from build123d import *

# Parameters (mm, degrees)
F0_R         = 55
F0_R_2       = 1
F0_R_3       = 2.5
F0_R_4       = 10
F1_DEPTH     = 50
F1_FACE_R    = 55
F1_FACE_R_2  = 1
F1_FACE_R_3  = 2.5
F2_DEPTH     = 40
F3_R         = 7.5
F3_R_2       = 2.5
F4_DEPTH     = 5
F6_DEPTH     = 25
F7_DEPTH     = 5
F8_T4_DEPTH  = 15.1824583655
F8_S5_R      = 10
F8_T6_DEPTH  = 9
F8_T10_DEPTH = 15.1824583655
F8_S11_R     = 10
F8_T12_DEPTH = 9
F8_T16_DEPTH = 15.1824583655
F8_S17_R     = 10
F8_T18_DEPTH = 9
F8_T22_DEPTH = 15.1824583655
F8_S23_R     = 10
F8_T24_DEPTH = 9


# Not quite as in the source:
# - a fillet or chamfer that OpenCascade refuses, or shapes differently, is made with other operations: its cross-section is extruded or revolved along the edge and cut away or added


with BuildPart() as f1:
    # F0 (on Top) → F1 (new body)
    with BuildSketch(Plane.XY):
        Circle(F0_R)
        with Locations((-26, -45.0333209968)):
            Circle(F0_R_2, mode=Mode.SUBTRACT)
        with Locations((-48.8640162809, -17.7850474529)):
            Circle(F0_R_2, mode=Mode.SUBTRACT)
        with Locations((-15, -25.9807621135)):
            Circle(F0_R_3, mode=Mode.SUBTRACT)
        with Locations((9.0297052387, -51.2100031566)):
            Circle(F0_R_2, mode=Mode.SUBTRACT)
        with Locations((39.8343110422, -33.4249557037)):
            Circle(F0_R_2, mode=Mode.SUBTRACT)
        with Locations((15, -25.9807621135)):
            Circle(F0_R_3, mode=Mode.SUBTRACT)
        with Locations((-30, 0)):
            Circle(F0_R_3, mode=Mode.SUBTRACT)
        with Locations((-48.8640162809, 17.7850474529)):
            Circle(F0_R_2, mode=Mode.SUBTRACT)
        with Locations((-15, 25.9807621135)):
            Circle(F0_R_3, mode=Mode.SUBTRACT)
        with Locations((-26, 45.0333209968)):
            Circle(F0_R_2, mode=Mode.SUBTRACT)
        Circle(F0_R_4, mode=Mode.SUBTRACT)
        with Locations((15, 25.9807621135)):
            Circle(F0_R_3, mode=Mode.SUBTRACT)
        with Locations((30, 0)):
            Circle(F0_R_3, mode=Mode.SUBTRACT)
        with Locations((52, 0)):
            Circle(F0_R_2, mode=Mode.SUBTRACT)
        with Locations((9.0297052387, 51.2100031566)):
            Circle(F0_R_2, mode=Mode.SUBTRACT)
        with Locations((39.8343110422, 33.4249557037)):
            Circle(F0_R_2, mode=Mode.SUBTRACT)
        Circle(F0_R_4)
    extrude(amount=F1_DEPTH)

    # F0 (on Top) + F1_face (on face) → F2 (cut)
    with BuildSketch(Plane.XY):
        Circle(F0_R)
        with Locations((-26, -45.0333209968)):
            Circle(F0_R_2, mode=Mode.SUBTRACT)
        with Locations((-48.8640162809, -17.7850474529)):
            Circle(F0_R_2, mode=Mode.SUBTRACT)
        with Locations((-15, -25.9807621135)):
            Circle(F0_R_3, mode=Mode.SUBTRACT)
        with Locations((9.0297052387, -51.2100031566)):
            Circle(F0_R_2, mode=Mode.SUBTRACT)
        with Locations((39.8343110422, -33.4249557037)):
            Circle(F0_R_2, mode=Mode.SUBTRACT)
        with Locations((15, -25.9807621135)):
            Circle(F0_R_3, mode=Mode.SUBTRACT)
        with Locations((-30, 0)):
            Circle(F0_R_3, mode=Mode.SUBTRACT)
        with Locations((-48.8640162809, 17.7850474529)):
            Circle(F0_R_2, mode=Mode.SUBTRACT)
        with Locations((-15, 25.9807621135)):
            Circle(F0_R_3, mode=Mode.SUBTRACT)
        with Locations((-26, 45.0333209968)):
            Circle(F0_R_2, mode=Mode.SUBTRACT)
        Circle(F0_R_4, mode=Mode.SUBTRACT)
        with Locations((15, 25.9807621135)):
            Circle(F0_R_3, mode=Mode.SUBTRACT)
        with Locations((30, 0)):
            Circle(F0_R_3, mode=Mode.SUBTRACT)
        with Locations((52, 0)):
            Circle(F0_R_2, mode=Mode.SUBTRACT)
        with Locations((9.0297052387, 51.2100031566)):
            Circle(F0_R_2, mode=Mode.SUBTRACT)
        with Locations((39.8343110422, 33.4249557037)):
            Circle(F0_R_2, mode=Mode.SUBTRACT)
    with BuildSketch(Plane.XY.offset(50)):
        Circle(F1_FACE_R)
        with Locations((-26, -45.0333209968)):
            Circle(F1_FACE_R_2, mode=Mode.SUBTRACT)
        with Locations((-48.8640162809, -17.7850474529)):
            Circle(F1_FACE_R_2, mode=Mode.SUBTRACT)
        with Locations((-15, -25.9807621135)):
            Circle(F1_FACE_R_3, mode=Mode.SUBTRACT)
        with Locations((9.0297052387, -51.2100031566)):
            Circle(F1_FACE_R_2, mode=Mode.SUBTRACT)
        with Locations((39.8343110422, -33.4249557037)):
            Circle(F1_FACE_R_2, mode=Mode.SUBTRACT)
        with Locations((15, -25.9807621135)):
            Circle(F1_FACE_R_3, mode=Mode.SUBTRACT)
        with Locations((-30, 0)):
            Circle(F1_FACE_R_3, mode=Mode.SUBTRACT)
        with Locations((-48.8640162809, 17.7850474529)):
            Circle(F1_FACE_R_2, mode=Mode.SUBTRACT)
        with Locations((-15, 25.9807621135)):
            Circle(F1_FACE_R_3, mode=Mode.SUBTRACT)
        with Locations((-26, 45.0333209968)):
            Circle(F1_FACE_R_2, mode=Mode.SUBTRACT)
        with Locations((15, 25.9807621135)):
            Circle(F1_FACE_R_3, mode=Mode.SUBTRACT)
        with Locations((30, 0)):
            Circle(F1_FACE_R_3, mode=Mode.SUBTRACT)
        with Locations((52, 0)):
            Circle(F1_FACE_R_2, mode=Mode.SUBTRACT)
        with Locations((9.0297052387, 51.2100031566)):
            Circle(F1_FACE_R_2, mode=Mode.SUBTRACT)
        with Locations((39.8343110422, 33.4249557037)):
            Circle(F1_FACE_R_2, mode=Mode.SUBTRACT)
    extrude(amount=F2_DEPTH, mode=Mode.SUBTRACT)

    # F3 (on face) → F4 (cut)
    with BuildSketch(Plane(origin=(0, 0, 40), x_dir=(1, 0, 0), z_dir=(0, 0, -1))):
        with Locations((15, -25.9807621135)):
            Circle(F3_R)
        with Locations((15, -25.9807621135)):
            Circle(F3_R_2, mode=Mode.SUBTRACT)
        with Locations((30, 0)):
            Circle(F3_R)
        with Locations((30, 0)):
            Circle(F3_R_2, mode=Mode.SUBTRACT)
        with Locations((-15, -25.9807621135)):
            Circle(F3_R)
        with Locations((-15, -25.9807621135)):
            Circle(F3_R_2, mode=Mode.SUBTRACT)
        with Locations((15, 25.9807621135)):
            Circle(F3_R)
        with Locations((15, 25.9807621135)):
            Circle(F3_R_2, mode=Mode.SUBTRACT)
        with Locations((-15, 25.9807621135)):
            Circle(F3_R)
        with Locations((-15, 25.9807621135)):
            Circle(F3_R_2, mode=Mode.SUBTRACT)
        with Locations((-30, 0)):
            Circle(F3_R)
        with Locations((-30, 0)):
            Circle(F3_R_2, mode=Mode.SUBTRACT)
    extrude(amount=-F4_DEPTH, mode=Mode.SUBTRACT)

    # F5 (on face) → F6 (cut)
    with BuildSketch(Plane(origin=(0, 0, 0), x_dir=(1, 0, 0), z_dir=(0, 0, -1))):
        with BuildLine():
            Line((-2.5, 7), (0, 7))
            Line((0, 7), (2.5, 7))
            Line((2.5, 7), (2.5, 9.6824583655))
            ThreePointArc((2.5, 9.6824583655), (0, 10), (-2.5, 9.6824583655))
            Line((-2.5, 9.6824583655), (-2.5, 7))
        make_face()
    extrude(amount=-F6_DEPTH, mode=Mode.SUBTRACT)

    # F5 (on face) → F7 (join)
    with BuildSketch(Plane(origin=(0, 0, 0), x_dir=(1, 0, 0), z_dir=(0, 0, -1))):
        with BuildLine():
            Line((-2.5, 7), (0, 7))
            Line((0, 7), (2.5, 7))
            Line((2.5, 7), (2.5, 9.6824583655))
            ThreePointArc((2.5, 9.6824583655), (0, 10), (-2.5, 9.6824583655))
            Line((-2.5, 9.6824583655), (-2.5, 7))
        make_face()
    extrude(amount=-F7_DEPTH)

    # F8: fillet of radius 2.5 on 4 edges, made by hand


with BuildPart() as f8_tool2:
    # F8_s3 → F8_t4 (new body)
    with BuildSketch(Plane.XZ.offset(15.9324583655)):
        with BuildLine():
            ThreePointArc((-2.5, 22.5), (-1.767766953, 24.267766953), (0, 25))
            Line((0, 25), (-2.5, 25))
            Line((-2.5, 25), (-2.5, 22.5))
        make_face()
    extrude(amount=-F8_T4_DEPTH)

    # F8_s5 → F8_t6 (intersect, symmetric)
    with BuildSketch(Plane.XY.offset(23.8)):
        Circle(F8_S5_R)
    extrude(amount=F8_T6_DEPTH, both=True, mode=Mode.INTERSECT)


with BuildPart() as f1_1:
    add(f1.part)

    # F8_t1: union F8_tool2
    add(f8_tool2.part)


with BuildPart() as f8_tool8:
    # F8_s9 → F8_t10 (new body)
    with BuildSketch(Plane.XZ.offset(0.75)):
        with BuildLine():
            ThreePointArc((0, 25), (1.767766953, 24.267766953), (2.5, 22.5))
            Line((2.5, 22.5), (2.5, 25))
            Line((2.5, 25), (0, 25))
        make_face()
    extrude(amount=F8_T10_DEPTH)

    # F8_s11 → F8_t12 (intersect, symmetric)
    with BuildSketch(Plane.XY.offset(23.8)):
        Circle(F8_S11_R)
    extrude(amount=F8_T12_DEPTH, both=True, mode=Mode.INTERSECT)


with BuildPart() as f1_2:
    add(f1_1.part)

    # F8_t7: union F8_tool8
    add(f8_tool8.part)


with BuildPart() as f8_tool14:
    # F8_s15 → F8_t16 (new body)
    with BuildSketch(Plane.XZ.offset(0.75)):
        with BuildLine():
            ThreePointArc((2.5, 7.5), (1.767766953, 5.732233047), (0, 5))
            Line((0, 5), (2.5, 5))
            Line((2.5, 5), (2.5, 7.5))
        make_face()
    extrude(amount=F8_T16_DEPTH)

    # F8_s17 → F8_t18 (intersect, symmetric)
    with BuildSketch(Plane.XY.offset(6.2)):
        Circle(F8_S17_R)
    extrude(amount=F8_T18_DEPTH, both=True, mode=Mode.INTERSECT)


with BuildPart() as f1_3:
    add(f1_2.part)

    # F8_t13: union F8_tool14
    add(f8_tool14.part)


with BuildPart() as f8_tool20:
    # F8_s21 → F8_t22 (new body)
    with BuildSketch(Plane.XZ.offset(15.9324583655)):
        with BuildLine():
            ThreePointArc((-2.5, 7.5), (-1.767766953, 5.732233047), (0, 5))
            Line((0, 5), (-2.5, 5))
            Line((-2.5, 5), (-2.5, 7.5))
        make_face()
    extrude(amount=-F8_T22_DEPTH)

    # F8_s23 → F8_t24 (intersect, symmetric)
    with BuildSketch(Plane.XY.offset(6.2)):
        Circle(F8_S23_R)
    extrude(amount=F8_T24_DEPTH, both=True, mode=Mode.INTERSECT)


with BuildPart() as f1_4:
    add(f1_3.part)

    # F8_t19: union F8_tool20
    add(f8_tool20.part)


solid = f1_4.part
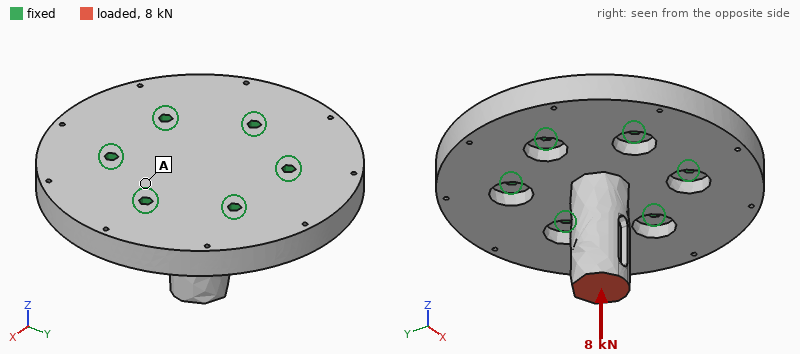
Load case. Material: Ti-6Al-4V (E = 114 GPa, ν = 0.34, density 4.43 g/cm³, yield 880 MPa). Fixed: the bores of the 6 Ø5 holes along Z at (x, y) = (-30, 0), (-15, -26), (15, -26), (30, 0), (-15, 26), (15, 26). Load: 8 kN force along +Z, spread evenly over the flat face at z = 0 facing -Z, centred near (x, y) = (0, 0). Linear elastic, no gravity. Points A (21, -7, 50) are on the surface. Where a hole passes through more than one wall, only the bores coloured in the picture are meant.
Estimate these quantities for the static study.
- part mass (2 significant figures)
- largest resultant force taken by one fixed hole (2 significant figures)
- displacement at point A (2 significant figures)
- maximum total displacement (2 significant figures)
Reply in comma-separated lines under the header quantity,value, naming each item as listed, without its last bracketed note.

quantity,value
part mass,450 g
largest resultant force taken by one fixed hole,1.9 kN
displacement at point A,6.8 µm
maximum total displacement,27 µm
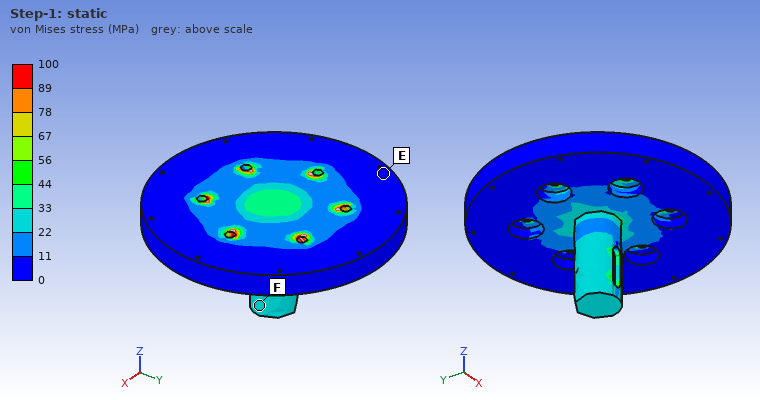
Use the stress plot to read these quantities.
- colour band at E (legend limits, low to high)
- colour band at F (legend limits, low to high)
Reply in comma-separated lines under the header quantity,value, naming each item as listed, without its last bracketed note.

quantity,value
colour band at E,0 to 11 MPa
colour band at F,22 to 33 MPa
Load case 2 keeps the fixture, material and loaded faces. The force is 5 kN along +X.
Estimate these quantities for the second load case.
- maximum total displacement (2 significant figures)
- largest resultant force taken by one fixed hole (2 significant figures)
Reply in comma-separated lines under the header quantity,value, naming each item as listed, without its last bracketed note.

quantity,value
maximum total displacement,0.23 mm
largest resultant force taken by one fixed hole,3.4 kN
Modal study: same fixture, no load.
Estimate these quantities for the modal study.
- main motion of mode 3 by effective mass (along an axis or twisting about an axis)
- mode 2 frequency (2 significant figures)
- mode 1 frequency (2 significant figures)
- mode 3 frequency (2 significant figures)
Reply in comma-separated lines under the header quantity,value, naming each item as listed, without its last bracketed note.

quantity,value
main motion of mode 3 by effective mass,along Z
mode 2 frequency,5800 Hz
mode 1 frequency,5800 Hz
mode 3 frequency,6900 Hz
